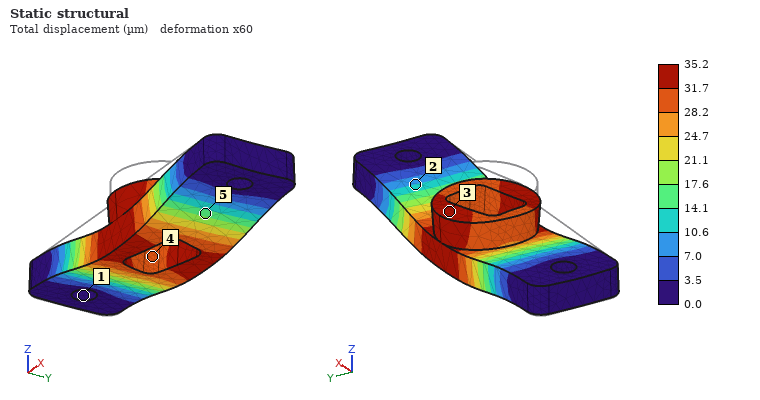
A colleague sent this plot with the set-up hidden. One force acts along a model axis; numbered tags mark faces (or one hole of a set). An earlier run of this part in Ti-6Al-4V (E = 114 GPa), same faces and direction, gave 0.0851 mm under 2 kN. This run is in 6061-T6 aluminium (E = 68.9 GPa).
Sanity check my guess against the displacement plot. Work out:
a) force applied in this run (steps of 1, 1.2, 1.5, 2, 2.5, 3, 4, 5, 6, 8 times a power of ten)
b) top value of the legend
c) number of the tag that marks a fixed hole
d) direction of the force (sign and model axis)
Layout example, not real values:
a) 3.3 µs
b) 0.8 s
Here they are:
a) 500 N
b) 35.2 µm
c) 1
d) -Z
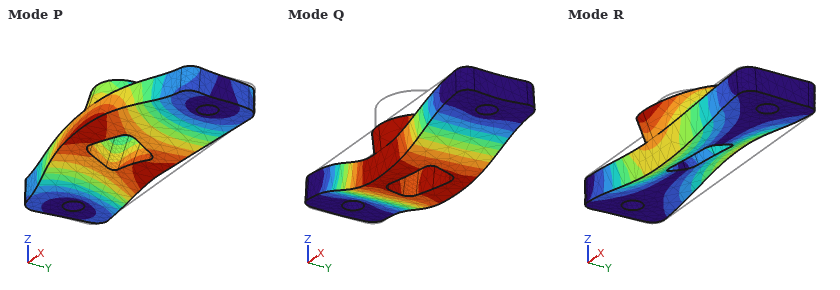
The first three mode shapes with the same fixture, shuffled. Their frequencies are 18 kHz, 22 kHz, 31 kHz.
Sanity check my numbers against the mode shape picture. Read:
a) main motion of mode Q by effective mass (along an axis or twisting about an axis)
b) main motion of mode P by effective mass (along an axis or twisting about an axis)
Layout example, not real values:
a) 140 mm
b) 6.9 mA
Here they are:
a) along Z
b) along Y
